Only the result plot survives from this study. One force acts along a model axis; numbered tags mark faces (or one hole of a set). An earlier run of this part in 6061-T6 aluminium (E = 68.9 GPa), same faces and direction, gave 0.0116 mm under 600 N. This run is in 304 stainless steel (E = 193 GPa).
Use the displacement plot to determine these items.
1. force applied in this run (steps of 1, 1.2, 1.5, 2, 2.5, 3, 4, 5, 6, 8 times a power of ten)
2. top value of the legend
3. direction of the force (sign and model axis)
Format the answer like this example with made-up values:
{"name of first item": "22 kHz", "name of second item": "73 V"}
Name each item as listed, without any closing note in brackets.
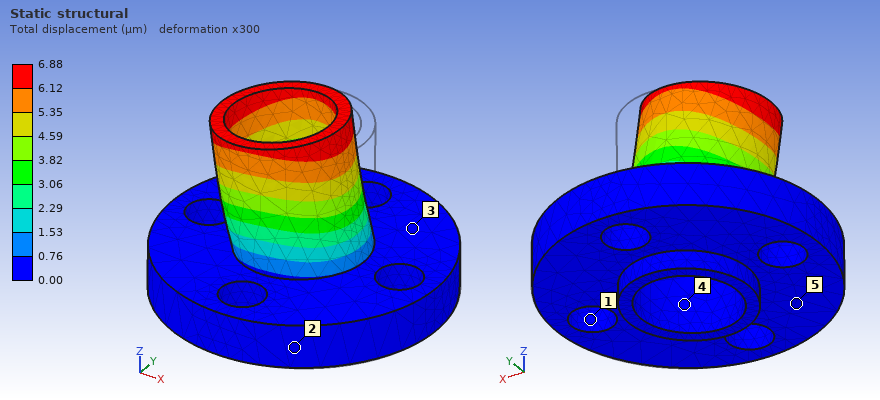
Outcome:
{"force applied in this run": "1 kN", "top value of the legend": "6.88 µm", "direction of the force": "-X"}
